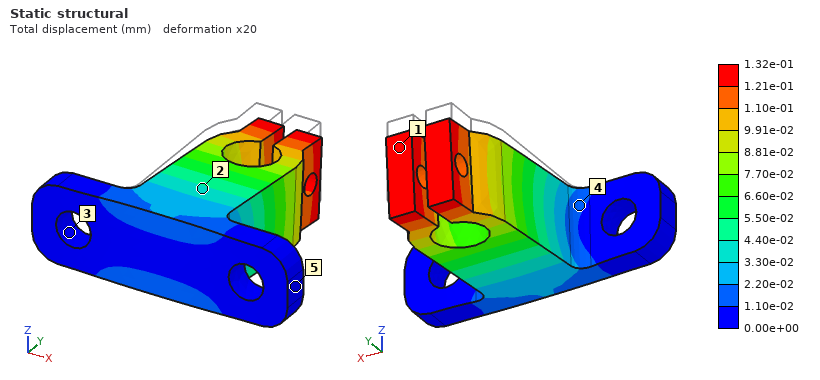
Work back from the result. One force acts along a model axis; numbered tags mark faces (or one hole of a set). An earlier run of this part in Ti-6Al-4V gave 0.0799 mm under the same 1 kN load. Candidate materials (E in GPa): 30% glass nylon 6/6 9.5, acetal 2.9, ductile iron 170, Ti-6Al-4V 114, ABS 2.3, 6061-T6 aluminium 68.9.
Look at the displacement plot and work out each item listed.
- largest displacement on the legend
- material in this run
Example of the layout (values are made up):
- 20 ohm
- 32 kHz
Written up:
- 1.32e-01 mm
- 6061-T6 aluminium
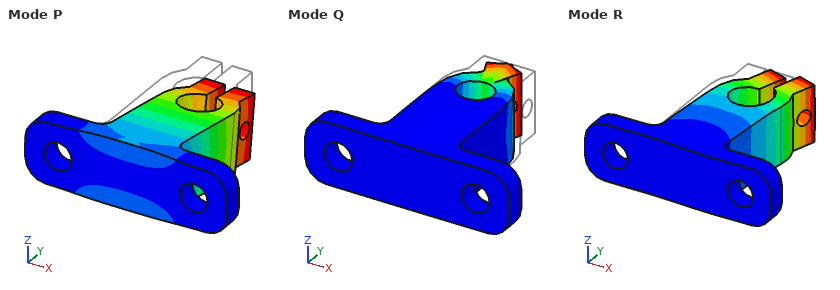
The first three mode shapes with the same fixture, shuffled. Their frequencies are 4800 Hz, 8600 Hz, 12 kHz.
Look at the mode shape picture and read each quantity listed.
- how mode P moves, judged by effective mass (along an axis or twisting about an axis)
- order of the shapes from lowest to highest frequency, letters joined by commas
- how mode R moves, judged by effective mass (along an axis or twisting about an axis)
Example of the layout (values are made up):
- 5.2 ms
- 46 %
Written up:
- along Z
- P, R, Q
- along X
